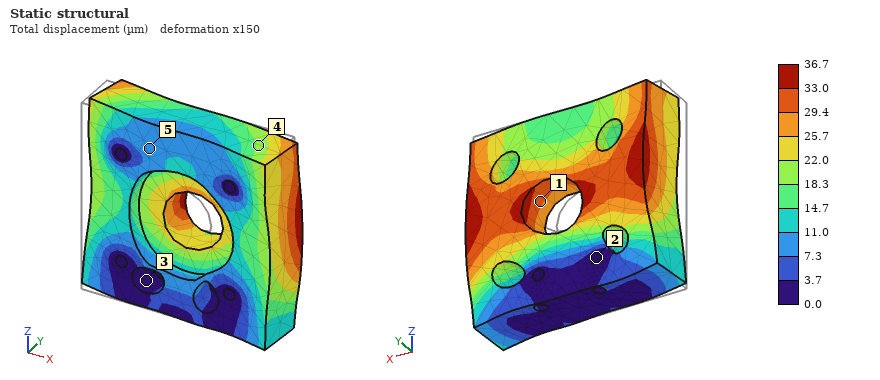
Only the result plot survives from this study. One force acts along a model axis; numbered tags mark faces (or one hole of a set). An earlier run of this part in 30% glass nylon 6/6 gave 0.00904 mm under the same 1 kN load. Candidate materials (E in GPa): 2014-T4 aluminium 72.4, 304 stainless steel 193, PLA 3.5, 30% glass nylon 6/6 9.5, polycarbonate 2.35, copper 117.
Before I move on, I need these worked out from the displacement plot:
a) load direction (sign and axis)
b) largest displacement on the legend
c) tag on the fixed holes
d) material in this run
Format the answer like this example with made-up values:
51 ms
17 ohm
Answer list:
+X
36.7 µm
2
polycarbonate
